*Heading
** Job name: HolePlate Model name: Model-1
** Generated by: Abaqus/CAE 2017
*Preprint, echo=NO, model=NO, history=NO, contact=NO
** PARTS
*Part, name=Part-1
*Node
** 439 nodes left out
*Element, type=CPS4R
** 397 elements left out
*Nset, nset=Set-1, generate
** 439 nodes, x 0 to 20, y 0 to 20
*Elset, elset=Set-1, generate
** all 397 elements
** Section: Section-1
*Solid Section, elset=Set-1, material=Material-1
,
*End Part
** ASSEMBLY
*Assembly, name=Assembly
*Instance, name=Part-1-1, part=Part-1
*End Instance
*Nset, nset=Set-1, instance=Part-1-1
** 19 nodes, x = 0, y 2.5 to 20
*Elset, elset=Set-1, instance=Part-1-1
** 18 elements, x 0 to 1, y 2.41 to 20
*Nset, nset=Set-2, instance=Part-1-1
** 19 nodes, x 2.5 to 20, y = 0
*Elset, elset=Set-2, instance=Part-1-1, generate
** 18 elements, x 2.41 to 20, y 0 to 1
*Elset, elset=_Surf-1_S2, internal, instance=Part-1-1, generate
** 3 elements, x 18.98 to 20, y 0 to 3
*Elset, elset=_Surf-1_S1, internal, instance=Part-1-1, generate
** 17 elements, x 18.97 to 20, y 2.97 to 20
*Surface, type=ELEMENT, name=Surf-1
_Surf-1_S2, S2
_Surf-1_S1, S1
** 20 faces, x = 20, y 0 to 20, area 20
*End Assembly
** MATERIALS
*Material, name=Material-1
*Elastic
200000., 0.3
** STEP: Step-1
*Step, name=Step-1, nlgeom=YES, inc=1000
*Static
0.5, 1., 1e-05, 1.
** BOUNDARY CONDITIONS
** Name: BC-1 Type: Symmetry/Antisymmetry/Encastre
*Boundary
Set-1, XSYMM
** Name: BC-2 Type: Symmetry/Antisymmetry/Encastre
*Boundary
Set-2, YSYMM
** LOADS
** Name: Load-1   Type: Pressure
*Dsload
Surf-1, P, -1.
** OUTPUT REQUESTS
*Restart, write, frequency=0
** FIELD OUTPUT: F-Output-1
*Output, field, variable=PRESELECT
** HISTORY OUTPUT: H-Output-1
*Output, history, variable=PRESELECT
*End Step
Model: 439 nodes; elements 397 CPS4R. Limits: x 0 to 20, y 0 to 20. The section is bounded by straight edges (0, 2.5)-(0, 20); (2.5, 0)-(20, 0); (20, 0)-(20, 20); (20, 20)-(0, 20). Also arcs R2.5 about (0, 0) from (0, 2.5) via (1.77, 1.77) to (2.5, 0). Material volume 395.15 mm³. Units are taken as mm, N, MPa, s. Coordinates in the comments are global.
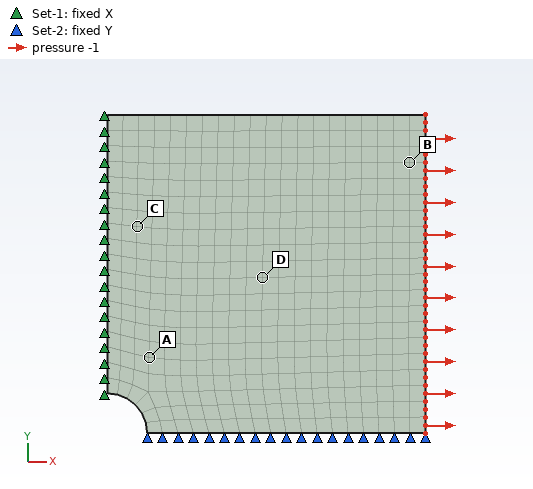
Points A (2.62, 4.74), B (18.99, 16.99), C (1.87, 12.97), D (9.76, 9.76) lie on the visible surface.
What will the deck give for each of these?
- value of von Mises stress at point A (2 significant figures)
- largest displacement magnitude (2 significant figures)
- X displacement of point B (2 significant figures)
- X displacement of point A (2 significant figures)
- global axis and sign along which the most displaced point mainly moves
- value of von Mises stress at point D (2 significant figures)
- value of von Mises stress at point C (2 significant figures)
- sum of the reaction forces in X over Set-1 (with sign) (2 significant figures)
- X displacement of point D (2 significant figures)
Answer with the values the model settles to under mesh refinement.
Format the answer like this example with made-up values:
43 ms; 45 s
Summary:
1.3 MPa; 1.1e-04 mm; 9.5e-05 mm; 1.6e-05 mm; +X; 1.1 MPa; 1.0 MPa; -20 N; 5.2e-05 mm
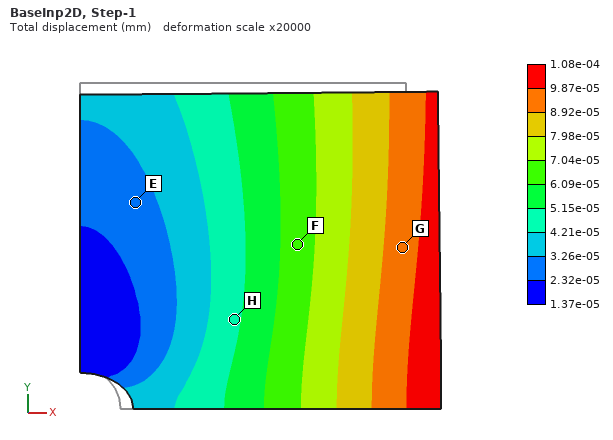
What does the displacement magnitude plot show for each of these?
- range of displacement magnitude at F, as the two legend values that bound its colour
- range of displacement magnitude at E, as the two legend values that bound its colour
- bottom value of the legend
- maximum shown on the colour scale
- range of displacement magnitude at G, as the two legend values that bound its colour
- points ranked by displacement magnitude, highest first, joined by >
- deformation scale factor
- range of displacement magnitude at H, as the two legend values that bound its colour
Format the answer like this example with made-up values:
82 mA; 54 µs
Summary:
6.09e-05 to 7.04e-05 mm; 2.32e-05 to 3.26e-05 mm; 1.37e-05 mm; 1.08e-04 mm; 8.92e-05 to 9.87e-05 mm; G > F > H > E; 20000; 4.21e-05 to 5.15e-05 mm
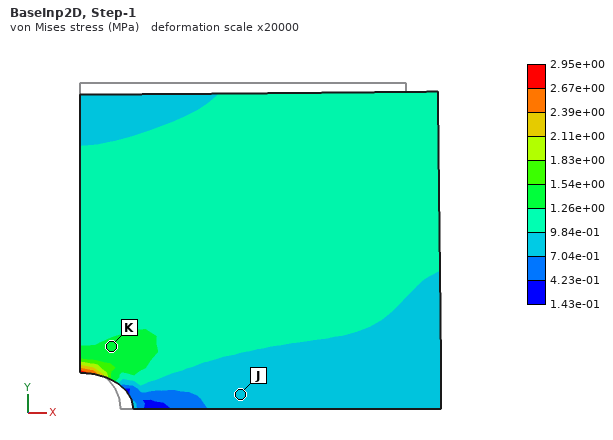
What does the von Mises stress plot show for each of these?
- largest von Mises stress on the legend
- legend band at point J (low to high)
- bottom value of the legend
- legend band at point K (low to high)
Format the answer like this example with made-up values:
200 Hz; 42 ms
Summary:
2.95e+00 MPa; 7.04e-01 to 9.84e-01 MPa; 1.43e-01 MPa; 1.26e+00 to 1.54e+00 MPa
